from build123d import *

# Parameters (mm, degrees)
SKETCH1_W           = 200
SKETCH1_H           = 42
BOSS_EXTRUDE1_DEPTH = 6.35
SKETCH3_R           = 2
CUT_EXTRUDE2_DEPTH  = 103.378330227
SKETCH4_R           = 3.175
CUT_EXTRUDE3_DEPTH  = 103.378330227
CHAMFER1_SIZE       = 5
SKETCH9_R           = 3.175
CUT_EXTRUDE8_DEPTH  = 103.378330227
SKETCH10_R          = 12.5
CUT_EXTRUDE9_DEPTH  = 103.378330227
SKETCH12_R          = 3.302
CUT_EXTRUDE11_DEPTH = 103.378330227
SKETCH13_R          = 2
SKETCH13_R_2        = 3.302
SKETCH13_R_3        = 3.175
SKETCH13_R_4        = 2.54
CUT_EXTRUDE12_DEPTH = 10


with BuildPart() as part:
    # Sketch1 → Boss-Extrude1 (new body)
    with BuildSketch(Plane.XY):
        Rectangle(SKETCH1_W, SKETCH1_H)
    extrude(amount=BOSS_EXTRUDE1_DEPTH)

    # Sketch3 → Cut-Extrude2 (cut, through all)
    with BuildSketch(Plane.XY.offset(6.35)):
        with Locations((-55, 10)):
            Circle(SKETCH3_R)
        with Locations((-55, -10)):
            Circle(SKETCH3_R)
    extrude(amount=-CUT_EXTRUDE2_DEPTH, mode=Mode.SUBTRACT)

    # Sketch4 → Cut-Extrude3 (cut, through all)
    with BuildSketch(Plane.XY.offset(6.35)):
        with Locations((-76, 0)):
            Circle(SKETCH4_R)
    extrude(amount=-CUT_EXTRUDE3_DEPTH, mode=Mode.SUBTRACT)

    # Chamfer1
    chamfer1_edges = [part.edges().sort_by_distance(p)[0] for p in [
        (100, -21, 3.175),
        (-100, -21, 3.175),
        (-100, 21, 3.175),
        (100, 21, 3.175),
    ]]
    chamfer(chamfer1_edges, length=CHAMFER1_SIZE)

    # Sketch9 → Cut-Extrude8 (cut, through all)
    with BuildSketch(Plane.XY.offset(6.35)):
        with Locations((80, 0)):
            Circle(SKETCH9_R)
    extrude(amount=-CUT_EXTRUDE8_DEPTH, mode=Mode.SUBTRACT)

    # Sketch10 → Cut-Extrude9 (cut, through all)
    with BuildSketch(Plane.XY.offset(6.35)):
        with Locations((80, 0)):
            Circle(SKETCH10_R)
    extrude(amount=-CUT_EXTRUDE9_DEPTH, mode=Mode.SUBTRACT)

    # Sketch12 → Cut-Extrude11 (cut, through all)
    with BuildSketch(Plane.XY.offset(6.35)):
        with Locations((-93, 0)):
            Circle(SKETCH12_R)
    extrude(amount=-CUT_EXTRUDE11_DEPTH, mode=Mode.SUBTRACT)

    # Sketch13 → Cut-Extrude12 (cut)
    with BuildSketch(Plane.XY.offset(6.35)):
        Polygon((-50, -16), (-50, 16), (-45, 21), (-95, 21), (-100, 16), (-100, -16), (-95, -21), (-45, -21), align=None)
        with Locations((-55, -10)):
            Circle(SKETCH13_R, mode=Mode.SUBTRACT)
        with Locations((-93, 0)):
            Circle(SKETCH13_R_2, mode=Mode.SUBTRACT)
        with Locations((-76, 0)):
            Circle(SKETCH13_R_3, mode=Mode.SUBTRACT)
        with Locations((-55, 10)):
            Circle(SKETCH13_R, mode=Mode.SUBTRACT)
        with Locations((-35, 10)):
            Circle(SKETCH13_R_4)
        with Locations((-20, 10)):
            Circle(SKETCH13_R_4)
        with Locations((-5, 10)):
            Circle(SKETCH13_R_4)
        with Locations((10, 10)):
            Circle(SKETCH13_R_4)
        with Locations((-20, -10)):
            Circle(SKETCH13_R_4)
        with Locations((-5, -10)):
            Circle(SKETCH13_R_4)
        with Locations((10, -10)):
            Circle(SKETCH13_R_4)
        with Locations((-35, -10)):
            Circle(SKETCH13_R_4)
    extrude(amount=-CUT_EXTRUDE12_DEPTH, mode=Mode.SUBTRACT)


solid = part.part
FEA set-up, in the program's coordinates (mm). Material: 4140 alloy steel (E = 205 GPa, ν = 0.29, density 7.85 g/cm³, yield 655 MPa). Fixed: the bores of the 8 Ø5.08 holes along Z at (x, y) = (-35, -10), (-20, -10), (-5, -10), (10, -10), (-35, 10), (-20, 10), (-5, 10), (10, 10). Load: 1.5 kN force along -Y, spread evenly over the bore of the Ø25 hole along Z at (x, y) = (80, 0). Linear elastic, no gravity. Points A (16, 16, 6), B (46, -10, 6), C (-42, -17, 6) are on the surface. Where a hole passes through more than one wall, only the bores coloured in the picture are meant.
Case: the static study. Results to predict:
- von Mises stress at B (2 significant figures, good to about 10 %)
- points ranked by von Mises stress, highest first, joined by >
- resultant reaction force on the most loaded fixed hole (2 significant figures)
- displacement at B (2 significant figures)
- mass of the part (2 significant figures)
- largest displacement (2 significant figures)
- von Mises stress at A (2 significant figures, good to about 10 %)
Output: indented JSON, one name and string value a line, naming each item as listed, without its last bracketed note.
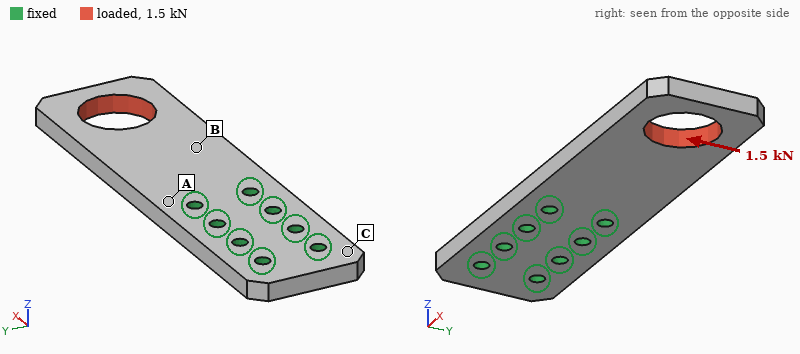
{
  "von Mises stress at B": "16 MPa",
  "points ranked by von Mises stress, highest first, joined by >": "A > B > C",
  "resultant reaction force on the most loaded fixed hole": "3.3 kN",
  "displacement at B": "13 µm",
  "mass of the part": "280 g",
  "largest displacement": "51 µm",
  "von Mises stress at A": "35 MPa"
}
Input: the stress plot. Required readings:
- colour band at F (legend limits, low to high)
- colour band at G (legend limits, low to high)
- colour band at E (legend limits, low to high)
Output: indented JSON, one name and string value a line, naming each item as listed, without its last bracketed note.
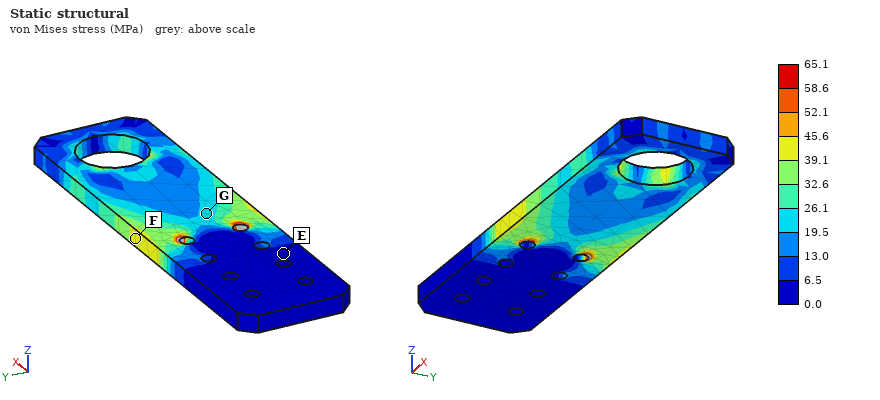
{
  "colour band at F": "39.1 to 45.6 MPa",
  "colour band at G": "19.5 to 26.1 MPa",
  "colour band at E": "0.0 to 6.5 MPa"
}
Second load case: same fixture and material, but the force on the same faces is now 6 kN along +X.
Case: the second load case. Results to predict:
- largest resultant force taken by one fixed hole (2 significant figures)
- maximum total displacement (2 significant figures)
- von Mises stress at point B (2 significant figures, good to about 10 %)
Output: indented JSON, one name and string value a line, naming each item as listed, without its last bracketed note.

{
  "largest resultant force taken by one fixed hole": "2.5 kN",
  "maximum total displacement": "17 µm",
  "von Mises stress at point B": "22 MPa"
}
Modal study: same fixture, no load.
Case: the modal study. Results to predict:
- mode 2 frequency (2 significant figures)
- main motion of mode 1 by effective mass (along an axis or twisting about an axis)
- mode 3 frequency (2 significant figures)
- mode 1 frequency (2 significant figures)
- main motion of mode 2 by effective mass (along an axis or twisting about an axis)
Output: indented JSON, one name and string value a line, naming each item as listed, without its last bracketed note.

{
  "mode 2 frequency": "2800 Hz",
  "main motion of mode 1 by effective mass": "along Z",
  "mode 3 frequency": "3700 Hz",
  "mode 1 frequency": "770 Hz",
  "main motion of mode 2 by effective mass": "twisting about X"
}
